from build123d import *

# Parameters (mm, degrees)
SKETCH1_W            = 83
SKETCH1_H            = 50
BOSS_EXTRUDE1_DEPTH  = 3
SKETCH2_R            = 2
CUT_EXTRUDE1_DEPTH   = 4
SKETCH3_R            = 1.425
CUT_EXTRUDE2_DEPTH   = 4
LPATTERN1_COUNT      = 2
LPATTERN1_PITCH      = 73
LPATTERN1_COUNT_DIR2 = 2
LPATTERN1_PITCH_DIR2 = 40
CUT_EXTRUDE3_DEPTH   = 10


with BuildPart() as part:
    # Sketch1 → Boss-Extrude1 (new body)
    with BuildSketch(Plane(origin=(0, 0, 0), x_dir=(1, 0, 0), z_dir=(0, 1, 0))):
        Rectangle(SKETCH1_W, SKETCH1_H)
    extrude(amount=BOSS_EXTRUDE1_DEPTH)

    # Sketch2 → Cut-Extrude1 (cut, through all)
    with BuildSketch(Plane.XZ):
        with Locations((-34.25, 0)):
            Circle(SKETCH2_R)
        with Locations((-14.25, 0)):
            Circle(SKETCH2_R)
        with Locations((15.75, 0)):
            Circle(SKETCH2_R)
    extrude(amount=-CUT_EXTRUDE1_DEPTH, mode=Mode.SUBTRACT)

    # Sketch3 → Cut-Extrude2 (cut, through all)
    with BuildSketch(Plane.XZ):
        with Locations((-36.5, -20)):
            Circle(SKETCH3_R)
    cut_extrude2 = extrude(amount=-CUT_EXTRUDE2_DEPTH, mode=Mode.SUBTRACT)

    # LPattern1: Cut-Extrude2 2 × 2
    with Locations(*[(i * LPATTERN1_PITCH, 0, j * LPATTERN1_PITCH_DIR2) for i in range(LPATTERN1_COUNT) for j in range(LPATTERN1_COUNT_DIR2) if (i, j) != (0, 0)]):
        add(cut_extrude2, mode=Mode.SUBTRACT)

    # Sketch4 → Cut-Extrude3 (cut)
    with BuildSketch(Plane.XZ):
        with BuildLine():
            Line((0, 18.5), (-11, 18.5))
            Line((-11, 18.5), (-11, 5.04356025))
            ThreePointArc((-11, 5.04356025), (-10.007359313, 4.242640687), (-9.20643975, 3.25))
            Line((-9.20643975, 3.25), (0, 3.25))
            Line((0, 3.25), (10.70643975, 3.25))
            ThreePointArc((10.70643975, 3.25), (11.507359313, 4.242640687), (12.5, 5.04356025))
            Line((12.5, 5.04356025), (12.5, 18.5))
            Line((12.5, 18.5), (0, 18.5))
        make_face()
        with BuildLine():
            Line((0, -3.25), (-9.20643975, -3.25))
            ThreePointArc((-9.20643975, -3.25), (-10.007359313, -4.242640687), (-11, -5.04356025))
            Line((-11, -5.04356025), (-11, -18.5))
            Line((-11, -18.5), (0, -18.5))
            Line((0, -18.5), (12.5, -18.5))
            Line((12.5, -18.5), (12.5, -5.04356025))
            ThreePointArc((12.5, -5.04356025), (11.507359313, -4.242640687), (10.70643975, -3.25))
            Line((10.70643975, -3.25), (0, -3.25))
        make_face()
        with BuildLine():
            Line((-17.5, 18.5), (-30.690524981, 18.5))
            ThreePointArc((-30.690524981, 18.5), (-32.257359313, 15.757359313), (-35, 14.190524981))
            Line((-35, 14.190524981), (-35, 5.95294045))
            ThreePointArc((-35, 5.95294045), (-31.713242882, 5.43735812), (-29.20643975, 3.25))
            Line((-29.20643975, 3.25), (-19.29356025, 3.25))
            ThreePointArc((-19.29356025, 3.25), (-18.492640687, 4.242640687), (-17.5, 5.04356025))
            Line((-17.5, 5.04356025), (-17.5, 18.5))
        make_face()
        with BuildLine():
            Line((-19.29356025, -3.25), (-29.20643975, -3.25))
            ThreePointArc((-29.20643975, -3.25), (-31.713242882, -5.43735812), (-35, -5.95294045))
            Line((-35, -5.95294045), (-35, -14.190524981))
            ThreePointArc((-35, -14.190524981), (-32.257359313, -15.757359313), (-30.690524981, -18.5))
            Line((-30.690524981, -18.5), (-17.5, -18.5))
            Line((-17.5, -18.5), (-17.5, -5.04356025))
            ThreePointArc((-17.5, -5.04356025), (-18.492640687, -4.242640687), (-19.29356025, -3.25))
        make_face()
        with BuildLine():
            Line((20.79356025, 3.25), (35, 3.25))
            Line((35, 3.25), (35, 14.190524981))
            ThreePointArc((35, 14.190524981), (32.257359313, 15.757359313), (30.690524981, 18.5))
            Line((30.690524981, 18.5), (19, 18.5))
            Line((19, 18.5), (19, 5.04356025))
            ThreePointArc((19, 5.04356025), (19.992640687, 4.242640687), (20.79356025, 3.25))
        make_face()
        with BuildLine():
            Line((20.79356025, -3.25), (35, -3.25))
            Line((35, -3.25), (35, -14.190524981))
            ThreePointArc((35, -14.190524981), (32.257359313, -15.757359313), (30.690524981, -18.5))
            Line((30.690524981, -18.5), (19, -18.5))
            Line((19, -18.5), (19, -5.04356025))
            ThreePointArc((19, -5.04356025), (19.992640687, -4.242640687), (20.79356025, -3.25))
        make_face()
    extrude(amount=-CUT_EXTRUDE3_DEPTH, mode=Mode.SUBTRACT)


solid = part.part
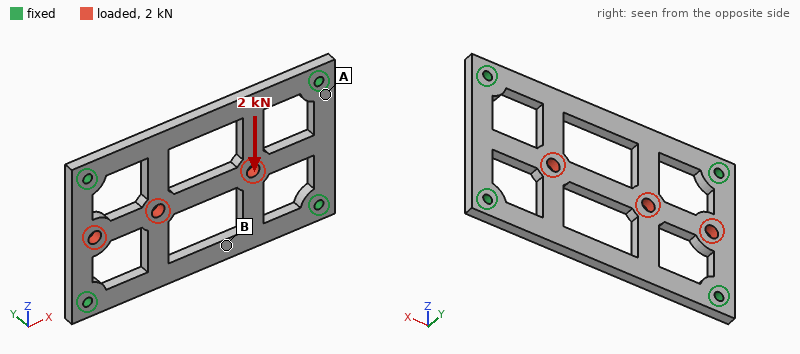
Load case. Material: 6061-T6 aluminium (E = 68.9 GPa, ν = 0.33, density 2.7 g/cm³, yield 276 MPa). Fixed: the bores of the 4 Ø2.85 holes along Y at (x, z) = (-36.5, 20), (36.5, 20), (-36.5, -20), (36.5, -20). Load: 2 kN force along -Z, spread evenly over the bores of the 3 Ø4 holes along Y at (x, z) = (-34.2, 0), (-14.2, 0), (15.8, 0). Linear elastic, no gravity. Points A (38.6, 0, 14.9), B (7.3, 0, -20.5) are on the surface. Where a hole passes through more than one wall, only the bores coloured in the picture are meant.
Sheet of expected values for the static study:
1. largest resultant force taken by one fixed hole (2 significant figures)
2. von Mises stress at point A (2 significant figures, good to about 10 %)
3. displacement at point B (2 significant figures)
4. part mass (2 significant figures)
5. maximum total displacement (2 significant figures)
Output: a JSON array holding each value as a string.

["690 N", "17 MPa", "51 µm", "20 g", "54 µm"]
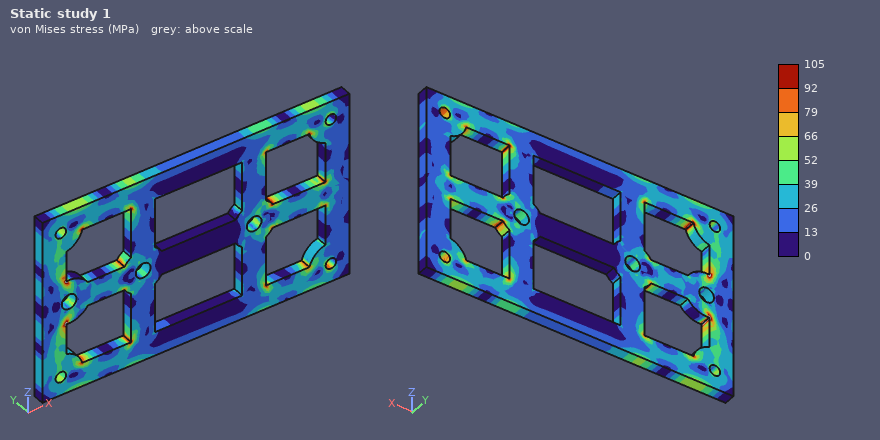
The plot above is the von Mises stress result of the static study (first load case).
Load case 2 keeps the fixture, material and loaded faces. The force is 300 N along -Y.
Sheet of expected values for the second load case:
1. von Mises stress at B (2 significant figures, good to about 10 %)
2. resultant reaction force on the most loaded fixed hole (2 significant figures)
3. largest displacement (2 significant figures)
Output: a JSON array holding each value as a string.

["22 MPa", "98 N", "0.15 mm"]
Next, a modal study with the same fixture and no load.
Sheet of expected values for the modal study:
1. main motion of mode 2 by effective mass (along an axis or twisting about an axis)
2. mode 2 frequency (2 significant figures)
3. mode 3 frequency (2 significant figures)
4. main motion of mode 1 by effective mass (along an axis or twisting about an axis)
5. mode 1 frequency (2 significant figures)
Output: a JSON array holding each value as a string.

["twisting about X", "3500 Hz", "5500 Hz", "along Y", "2400 Hz"]
